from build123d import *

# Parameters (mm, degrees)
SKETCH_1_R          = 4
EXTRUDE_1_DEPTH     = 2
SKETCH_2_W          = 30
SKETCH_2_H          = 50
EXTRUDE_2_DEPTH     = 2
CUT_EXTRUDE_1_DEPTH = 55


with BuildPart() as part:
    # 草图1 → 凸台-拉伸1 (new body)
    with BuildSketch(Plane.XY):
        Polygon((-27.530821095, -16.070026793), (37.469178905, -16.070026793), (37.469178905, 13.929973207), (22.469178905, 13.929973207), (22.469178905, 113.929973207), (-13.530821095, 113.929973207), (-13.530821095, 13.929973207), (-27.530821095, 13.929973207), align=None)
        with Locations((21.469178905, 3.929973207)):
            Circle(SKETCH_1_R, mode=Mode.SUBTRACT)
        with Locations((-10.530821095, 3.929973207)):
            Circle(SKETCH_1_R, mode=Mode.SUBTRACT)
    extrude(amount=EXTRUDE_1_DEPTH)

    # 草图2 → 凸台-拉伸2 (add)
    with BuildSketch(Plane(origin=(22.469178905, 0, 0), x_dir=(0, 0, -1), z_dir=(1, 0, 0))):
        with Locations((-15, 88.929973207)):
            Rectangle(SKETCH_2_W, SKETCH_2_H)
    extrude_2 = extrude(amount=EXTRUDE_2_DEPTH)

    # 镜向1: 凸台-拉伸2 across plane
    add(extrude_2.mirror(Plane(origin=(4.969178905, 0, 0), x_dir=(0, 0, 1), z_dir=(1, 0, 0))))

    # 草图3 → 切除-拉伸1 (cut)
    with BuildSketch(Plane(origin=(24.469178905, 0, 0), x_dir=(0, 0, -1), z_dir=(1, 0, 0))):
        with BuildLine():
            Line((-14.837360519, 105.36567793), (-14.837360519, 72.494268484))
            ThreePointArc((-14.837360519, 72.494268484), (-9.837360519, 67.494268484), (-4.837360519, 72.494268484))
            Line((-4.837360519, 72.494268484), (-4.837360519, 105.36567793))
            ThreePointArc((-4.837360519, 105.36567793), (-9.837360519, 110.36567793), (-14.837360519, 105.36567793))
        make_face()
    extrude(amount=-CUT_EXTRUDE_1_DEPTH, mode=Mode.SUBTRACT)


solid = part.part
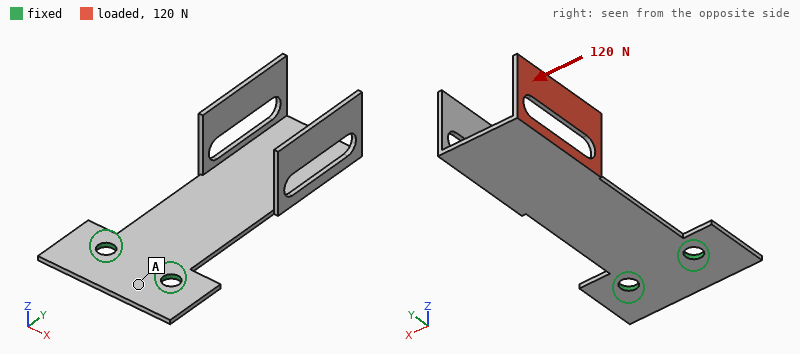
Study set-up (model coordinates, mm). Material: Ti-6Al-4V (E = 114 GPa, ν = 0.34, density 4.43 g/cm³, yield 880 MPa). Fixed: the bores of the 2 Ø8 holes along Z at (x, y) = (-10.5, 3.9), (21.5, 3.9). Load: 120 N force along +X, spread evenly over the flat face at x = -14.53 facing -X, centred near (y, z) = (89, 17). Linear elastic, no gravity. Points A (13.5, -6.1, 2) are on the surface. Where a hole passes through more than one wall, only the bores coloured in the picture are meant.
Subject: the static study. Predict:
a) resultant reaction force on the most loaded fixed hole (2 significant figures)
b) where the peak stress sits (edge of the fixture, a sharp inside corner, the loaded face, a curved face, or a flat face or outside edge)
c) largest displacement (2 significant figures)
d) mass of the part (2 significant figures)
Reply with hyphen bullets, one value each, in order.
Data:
- 320 N
- a curved face
- 1.7 mm
- 67 g
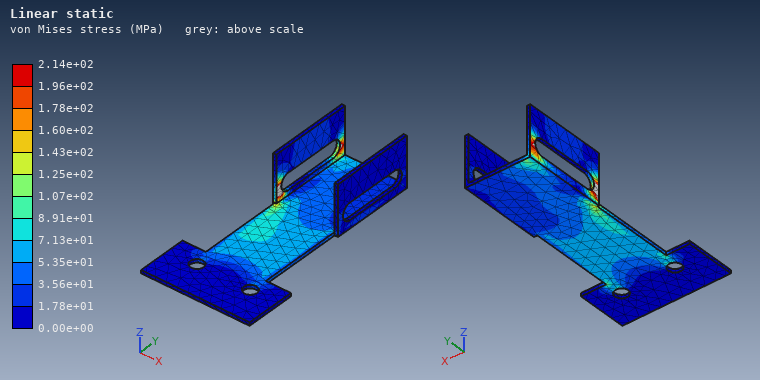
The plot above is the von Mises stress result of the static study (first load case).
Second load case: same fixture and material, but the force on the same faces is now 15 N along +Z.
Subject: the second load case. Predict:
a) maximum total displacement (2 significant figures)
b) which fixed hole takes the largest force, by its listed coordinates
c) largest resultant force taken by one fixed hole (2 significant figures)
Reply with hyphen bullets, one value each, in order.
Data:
- 1.6 mm
- (-10.5, 3.9)
- 18 N
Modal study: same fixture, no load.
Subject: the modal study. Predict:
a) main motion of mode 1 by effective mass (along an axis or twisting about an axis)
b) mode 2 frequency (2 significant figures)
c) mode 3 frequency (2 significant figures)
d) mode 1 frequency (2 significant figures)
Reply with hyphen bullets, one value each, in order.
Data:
- along Z
- 330 Hz
- 690 Hz
- 98 Hz
